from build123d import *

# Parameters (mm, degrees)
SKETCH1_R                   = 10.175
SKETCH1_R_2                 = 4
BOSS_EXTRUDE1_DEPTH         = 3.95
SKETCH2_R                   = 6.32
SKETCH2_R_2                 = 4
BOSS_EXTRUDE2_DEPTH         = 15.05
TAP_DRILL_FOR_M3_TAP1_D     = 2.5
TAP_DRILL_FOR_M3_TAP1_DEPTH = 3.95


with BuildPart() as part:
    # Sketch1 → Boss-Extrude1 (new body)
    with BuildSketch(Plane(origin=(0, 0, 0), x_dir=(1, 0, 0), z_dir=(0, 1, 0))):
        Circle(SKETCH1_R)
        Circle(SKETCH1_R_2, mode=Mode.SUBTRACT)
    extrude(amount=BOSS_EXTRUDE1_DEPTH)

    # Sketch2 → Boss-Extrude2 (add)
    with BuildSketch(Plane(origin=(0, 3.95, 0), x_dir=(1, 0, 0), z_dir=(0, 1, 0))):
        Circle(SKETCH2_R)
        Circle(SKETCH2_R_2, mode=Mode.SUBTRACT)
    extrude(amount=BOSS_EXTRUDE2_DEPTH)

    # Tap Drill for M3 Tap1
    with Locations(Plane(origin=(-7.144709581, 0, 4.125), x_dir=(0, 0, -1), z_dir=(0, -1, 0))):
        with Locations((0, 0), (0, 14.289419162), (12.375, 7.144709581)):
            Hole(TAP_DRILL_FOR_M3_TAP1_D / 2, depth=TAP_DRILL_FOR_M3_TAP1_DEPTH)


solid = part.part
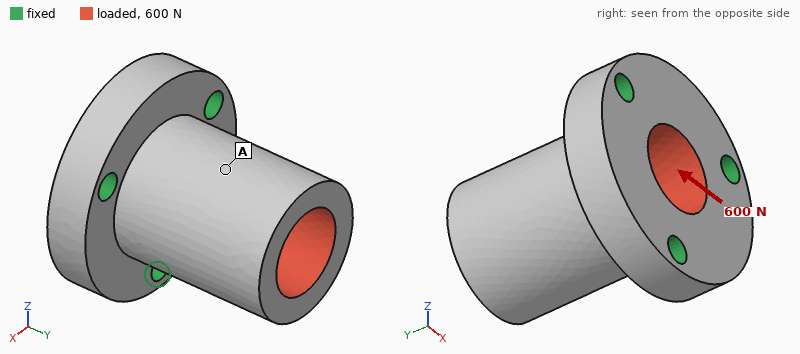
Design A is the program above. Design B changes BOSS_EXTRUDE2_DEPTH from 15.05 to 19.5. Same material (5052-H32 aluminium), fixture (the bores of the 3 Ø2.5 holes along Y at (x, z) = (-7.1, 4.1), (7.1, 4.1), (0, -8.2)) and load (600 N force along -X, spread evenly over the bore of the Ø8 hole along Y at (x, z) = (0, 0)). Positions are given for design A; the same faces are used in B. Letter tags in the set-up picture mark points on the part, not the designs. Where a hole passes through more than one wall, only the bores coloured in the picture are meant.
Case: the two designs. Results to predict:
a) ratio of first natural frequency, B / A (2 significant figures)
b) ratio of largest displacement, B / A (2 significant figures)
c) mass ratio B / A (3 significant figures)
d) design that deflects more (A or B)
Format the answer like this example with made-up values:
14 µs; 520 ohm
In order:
0.70; 1.7; 1.15; B
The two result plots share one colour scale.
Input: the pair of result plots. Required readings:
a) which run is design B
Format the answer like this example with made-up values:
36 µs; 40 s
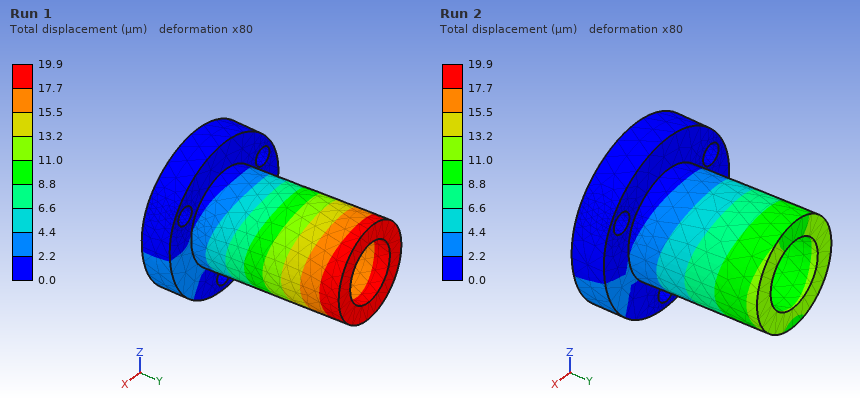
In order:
Run 1
